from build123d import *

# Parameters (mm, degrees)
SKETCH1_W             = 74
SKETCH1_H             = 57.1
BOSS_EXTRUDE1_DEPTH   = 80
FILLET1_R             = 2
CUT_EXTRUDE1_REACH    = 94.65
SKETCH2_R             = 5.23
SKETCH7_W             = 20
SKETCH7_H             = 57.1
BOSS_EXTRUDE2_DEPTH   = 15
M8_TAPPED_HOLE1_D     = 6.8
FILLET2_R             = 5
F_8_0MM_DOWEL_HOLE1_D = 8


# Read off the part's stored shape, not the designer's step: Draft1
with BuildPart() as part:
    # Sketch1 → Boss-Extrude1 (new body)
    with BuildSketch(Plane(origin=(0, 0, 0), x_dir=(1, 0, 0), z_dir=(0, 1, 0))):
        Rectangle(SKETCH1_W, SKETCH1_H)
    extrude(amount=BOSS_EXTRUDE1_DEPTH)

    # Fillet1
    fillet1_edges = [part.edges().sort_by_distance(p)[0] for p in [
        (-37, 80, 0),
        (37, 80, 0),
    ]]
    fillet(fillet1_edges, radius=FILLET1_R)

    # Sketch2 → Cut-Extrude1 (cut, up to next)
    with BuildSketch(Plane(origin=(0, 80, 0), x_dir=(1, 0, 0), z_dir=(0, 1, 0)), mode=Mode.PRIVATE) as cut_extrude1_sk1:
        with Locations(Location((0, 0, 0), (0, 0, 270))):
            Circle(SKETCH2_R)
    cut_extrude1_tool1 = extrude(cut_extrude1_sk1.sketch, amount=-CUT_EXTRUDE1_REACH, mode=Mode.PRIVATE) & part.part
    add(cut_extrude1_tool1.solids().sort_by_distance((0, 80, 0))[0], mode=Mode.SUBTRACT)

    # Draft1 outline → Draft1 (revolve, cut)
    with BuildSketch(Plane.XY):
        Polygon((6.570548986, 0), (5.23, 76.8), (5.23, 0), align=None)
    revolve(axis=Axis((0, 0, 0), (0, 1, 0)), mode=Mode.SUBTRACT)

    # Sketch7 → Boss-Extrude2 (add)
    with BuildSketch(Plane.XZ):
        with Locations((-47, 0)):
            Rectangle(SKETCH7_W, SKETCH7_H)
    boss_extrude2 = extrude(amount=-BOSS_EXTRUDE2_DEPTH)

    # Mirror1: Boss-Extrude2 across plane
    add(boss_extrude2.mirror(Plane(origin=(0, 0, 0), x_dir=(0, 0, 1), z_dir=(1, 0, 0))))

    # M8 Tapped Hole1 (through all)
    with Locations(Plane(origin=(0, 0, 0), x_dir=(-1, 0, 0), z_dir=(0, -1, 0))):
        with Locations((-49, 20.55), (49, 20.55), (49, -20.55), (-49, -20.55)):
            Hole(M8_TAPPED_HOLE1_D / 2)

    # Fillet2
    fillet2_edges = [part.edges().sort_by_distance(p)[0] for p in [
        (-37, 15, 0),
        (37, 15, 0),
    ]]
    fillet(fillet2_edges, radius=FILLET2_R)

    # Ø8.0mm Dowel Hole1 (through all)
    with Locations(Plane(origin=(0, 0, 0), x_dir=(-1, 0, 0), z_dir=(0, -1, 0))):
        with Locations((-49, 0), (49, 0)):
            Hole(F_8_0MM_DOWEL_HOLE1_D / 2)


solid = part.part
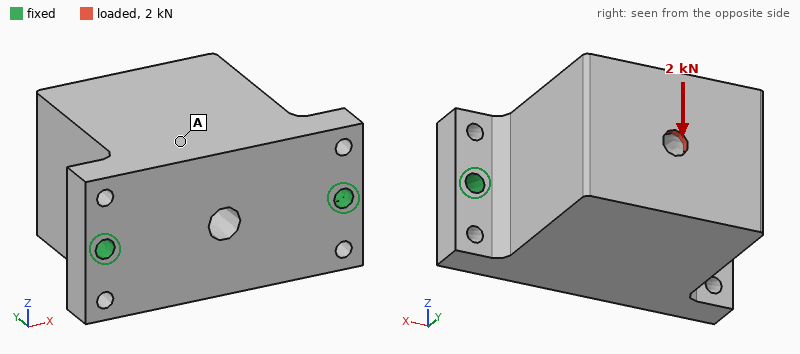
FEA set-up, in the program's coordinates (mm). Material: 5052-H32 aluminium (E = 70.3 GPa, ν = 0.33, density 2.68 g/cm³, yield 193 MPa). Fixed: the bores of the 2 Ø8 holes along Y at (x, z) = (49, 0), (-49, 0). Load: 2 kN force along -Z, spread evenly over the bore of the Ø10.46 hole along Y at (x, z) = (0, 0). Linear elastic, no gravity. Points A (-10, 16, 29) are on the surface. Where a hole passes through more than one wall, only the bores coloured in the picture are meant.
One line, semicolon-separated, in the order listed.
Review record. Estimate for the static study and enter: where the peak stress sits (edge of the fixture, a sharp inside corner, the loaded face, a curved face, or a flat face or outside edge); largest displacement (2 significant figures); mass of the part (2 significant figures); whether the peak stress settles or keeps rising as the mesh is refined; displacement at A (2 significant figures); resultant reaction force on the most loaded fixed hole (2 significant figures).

edge of the fixture; 89 µm; 970 g; keeps rising; 33 µm; 1.0 kN
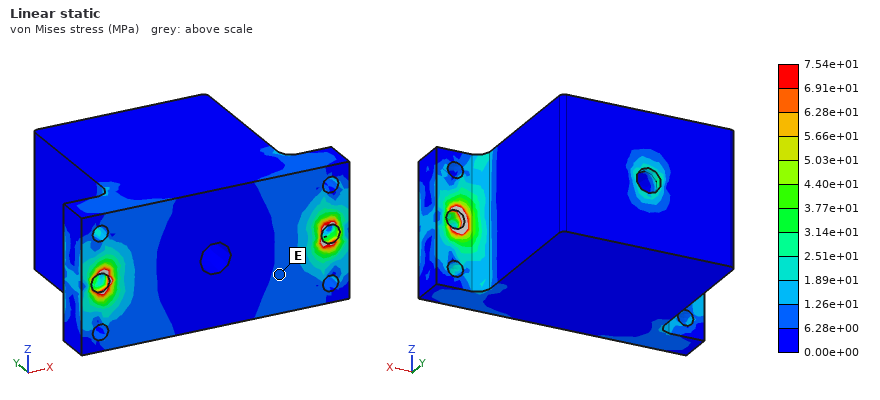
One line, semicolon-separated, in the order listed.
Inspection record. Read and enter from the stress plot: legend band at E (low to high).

6.28e+00 to 1.26e+01 MPa
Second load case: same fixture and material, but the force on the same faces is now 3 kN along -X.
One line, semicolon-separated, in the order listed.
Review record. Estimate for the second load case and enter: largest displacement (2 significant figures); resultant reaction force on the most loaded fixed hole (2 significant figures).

15 µm; 2.8 kN
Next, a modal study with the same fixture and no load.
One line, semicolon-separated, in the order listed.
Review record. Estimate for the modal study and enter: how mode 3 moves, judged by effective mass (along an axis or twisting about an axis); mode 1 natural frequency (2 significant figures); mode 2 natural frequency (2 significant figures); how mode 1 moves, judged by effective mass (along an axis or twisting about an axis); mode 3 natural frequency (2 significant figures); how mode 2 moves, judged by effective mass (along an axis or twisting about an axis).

along Y; 1400 Hz; 4400 Hz; along Z; 4800 Hz; along X
